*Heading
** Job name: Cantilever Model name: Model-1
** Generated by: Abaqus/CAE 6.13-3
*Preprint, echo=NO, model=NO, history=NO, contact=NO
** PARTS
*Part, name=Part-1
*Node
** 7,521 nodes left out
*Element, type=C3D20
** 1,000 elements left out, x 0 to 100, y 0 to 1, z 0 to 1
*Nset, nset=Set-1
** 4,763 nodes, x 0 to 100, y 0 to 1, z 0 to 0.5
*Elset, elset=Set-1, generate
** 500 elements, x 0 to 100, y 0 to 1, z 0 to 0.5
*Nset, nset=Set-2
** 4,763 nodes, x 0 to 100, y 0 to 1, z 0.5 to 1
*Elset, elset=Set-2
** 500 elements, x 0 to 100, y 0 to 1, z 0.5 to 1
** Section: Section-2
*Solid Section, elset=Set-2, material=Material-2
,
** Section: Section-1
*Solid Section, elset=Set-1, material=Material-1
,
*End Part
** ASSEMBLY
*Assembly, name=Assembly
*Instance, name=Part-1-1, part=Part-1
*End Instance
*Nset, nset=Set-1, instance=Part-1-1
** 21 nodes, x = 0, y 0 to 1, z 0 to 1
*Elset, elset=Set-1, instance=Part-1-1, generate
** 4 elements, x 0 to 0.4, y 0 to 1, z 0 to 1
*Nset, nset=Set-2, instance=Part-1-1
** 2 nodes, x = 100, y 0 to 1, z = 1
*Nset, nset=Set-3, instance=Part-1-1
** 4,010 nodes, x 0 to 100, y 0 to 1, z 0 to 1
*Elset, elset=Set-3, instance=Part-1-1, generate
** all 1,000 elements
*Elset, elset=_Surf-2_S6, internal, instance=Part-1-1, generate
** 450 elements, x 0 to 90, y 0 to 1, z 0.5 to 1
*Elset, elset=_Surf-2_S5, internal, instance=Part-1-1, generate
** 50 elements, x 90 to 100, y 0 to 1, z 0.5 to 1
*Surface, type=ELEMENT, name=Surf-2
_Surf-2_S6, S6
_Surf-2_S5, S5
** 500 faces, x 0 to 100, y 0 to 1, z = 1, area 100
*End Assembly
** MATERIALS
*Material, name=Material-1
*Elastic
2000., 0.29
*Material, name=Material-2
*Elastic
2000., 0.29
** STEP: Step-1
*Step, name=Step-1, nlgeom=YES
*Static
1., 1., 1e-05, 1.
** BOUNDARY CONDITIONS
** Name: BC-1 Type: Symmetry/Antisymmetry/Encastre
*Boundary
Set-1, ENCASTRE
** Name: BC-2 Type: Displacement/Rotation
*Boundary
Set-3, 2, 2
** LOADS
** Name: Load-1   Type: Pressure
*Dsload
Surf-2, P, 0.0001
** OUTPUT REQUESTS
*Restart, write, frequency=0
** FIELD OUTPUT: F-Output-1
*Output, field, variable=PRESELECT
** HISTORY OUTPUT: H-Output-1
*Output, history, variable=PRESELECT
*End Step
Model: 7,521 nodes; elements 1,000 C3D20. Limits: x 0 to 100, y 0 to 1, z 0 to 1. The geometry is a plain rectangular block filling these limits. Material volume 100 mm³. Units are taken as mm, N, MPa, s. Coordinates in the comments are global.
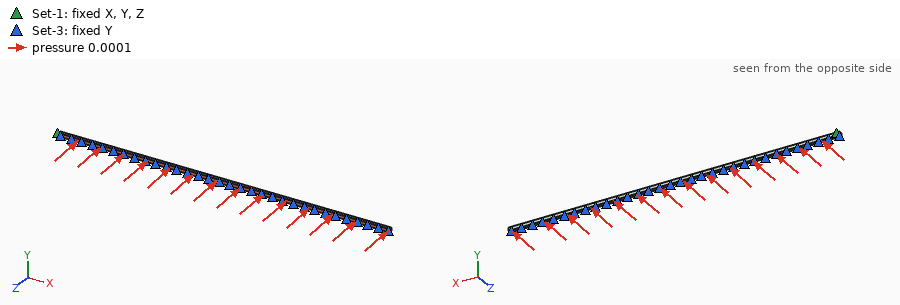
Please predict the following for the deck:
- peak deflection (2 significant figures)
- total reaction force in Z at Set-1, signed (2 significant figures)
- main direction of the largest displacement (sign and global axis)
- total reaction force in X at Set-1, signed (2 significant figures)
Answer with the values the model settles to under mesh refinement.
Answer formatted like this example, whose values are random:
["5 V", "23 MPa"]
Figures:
["6.9 mm", "0.010 N", "-Z", "6.9e-04 N"]
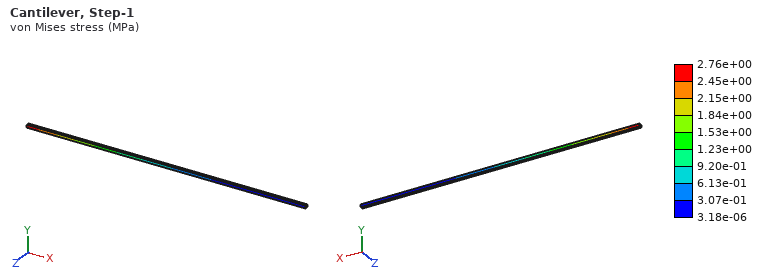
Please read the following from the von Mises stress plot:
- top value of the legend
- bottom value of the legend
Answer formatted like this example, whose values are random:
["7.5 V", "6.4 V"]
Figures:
["2.76e+00 MPa", "3.18e-06 MPa"]
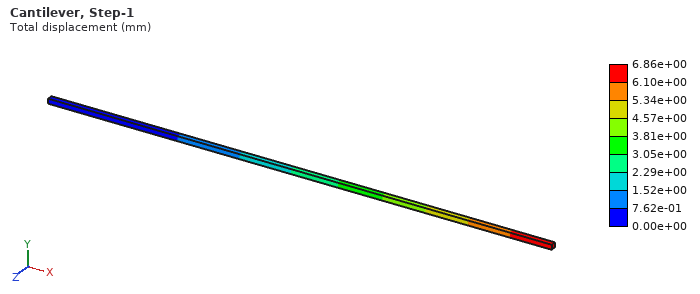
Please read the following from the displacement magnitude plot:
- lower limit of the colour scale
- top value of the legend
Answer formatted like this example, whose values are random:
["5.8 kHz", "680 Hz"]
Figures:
["0.00e+00 mm", "6.86e+00 mm"]
